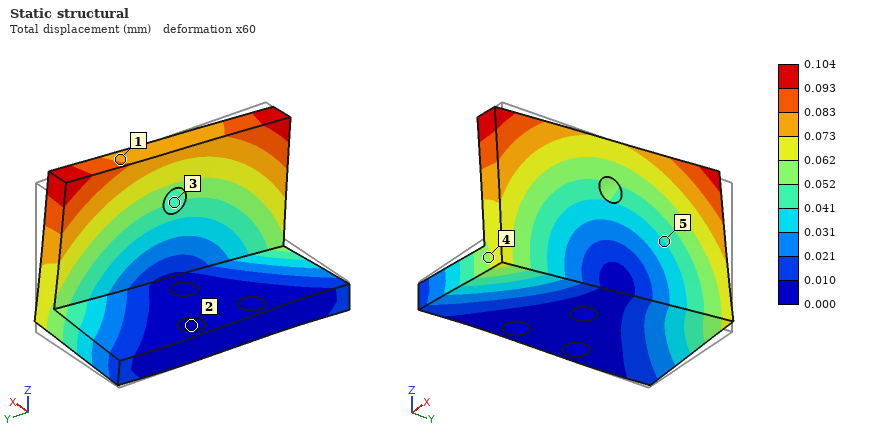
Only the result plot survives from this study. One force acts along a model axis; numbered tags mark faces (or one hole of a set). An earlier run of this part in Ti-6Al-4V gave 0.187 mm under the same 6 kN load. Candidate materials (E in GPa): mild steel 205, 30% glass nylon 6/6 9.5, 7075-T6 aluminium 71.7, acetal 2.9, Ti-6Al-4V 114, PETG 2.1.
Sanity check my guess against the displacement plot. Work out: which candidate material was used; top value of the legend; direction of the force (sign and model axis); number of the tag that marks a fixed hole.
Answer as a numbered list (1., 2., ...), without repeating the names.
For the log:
1. mild steel
2. 0.104 mm
3. -Y
4. 2
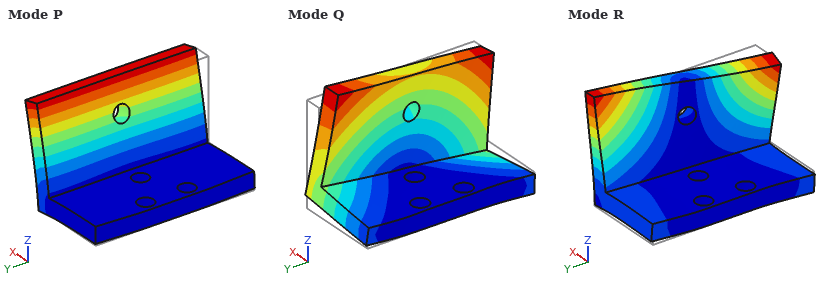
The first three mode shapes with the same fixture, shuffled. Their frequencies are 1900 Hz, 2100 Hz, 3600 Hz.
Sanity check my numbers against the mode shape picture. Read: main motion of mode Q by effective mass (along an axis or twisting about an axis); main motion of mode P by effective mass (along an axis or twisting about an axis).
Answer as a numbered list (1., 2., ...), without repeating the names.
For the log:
1. along Y
2. along X
